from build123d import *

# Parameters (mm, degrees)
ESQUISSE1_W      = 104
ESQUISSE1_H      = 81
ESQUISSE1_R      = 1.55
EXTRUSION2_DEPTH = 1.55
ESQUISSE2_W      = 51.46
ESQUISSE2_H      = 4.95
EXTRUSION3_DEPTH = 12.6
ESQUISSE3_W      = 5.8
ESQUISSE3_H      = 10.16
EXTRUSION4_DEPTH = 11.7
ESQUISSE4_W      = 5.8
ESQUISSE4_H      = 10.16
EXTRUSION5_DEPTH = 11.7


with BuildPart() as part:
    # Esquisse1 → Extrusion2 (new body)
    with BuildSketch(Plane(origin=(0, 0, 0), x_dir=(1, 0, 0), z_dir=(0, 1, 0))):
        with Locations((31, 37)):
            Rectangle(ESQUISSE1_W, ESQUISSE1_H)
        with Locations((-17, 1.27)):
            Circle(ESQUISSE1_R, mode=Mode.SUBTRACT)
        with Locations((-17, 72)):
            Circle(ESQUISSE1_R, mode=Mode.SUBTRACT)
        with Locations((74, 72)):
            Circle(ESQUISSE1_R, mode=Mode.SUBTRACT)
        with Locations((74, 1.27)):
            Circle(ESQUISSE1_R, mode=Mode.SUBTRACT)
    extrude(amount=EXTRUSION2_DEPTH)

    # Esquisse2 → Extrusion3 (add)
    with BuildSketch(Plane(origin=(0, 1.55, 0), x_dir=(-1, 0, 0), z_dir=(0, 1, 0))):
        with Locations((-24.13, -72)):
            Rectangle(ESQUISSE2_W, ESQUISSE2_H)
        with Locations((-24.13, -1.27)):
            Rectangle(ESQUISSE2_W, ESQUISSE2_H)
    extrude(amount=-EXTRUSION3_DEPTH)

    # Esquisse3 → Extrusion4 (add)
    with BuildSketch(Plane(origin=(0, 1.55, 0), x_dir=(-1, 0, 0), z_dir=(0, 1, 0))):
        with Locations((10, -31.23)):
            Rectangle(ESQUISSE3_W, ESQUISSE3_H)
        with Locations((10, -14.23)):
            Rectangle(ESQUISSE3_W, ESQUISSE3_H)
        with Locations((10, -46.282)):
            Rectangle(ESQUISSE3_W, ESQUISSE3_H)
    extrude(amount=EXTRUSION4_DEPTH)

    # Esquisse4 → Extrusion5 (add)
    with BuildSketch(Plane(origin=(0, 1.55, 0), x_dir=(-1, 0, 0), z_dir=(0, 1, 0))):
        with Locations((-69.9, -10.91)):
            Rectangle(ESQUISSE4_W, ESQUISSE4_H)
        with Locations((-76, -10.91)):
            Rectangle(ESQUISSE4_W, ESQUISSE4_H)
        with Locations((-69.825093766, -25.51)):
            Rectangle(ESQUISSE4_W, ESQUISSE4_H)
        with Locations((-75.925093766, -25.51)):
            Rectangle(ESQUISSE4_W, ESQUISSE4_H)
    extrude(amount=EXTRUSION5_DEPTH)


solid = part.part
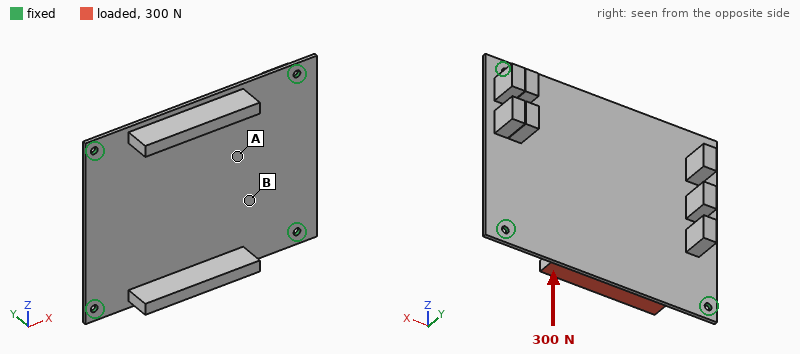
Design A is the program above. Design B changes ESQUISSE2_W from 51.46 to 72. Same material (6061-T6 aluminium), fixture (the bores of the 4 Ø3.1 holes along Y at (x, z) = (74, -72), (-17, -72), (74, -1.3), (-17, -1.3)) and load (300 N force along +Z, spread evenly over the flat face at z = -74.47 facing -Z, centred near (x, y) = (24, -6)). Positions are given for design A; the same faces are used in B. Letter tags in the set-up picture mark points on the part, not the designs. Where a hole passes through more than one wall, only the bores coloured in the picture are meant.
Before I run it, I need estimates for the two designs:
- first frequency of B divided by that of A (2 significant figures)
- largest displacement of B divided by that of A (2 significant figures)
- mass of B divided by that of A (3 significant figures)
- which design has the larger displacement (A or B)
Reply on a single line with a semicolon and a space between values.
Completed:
1.1; 0.56; 1.10; A
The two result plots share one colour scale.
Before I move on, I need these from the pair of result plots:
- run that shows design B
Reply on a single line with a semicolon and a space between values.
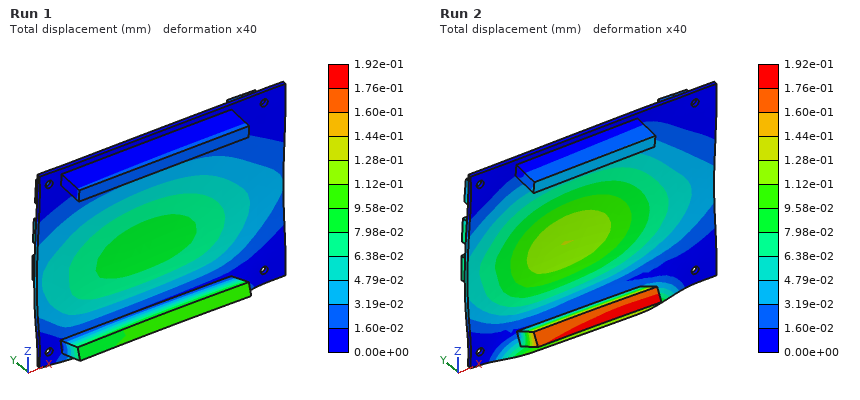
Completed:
Run 1
